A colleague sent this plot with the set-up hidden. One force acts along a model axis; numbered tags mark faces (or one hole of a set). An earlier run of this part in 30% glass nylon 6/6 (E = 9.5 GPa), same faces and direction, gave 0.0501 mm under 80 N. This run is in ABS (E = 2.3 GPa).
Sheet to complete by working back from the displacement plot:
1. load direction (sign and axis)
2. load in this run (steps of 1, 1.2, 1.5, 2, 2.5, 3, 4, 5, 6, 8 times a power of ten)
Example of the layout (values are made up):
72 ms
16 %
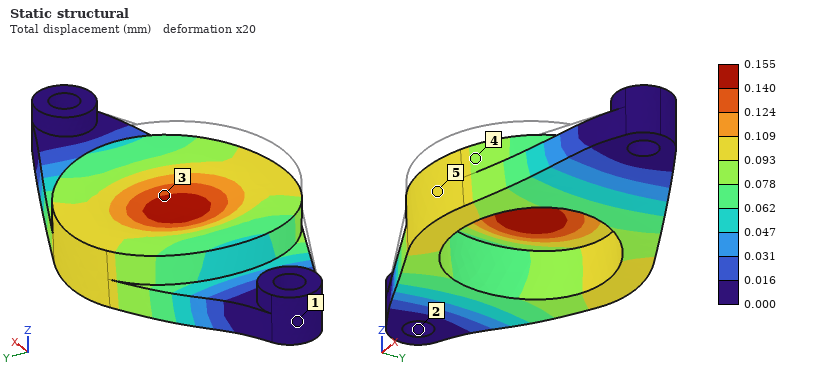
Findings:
-Z
60 N
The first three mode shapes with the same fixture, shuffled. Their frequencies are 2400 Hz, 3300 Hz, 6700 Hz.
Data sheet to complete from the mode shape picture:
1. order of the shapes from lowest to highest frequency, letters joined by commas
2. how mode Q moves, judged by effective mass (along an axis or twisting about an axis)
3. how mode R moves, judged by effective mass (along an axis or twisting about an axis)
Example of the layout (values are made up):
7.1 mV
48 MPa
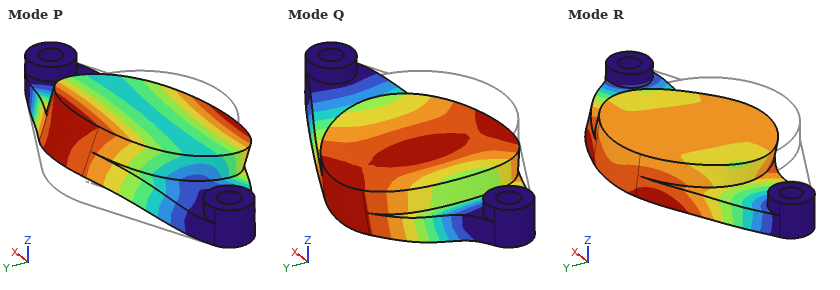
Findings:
P, Q, R
along Z
along Y
